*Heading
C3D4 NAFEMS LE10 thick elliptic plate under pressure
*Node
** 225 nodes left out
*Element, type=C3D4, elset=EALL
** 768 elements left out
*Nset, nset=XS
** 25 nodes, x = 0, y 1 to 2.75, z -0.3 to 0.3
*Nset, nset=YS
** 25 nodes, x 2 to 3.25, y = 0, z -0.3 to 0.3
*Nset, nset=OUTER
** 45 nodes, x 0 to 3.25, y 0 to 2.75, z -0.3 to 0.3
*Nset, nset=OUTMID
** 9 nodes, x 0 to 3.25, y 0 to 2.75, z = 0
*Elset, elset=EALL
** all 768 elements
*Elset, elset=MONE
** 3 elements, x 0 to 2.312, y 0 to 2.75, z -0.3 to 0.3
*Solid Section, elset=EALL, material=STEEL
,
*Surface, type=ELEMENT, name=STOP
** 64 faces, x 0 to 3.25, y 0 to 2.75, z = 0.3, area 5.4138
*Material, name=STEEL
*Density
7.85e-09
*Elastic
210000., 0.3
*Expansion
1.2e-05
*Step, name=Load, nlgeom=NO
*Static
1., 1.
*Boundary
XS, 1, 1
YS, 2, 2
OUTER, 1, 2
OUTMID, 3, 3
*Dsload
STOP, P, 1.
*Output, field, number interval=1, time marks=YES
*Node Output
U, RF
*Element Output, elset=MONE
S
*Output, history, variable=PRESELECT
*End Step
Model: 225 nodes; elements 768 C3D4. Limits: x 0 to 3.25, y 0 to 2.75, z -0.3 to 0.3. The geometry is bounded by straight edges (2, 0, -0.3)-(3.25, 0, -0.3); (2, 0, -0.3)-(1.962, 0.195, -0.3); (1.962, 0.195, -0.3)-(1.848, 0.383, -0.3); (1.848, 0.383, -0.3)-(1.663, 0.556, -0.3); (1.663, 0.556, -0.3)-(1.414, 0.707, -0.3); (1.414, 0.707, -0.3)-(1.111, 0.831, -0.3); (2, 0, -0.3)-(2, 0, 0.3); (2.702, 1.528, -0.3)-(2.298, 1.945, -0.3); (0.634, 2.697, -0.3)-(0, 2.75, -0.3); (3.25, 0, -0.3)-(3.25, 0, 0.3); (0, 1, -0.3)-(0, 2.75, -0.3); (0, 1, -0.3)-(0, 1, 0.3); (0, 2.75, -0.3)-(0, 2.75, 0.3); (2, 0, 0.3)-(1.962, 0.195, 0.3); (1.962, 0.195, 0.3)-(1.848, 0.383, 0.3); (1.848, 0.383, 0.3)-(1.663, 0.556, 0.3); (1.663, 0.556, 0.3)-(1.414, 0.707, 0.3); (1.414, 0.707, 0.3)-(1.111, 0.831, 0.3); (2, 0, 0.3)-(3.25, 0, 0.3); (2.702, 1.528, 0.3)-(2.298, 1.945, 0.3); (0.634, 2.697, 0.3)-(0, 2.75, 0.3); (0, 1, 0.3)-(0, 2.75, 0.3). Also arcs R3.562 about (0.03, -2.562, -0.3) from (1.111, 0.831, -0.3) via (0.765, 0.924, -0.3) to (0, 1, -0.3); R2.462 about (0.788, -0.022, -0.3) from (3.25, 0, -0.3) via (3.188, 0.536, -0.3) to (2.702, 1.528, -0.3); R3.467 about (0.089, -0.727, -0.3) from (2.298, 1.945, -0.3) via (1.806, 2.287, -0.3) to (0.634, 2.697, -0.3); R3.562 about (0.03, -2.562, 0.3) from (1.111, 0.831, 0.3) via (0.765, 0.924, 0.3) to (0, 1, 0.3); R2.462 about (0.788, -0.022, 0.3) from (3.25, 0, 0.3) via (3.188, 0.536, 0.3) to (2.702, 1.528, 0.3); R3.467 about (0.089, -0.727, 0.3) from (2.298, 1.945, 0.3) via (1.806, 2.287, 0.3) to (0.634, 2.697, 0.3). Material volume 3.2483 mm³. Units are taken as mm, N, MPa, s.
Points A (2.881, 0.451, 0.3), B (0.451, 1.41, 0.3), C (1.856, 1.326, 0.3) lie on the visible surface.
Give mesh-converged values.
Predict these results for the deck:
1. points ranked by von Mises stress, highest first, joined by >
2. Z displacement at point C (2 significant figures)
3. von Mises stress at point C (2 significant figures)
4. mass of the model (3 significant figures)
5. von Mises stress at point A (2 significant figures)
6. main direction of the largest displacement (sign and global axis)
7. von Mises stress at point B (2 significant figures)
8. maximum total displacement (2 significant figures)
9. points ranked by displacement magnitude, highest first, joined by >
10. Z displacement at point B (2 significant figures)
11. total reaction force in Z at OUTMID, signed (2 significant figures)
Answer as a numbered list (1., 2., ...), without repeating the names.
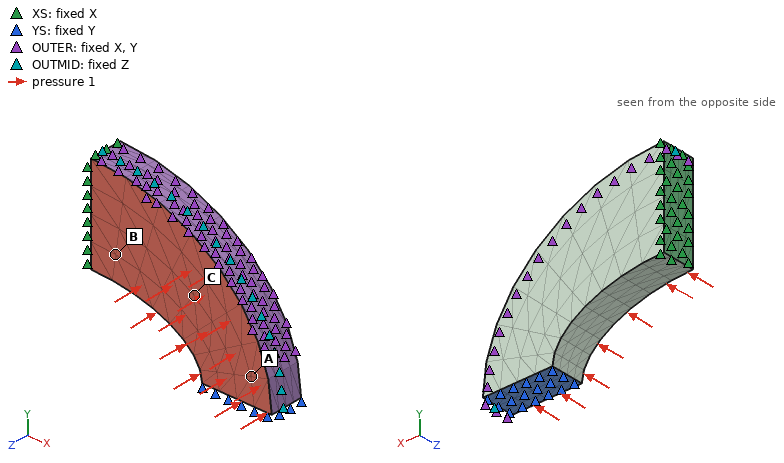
1. A > C > B
2. -6.1e-05 mm
3. 4.7 MPa
4. 2.55e-05 kg
5. 7.1 MPa
6. -Z
7. 3.9 MPa
8. 2.0e-04 mm
9. B > C > A
10. -1.4e-04 mm
11. 5.4 N
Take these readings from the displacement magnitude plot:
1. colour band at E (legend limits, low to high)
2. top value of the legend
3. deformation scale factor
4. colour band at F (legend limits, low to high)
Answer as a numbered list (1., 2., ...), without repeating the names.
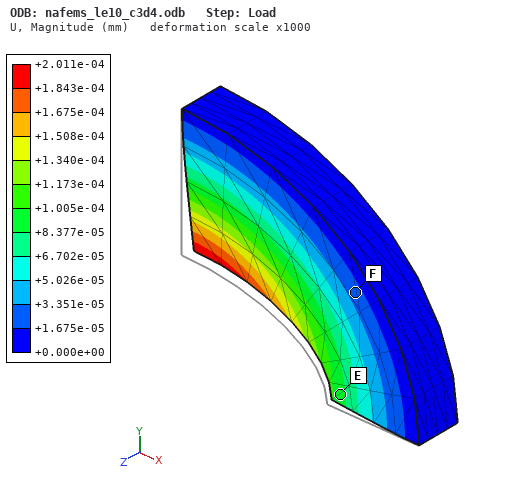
1. +8.377e-05 to +1.005e-04 mm
2. +2.011e-04 mm
3. 1000
4. +1.675e-05 to +3.351e-05 mm
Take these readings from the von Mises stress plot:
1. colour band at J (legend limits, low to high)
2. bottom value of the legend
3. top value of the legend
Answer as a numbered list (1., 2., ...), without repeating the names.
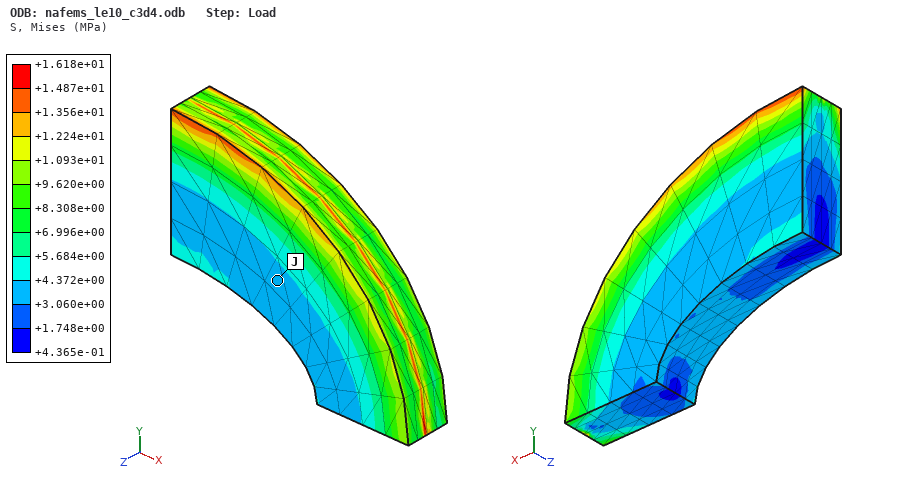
1. +3.060e+00 to +4.372e+00 MPa
2. +4.365e-01 MPa
3. +1.618e+01 MPa
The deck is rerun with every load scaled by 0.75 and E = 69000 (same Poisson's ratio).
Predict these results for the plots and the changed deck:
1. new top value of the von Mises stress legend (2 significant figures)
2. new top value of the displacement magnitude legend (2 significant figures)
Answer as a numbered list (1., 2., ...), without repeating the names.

1. 12 MPa
2. 4.6e-04 mm
